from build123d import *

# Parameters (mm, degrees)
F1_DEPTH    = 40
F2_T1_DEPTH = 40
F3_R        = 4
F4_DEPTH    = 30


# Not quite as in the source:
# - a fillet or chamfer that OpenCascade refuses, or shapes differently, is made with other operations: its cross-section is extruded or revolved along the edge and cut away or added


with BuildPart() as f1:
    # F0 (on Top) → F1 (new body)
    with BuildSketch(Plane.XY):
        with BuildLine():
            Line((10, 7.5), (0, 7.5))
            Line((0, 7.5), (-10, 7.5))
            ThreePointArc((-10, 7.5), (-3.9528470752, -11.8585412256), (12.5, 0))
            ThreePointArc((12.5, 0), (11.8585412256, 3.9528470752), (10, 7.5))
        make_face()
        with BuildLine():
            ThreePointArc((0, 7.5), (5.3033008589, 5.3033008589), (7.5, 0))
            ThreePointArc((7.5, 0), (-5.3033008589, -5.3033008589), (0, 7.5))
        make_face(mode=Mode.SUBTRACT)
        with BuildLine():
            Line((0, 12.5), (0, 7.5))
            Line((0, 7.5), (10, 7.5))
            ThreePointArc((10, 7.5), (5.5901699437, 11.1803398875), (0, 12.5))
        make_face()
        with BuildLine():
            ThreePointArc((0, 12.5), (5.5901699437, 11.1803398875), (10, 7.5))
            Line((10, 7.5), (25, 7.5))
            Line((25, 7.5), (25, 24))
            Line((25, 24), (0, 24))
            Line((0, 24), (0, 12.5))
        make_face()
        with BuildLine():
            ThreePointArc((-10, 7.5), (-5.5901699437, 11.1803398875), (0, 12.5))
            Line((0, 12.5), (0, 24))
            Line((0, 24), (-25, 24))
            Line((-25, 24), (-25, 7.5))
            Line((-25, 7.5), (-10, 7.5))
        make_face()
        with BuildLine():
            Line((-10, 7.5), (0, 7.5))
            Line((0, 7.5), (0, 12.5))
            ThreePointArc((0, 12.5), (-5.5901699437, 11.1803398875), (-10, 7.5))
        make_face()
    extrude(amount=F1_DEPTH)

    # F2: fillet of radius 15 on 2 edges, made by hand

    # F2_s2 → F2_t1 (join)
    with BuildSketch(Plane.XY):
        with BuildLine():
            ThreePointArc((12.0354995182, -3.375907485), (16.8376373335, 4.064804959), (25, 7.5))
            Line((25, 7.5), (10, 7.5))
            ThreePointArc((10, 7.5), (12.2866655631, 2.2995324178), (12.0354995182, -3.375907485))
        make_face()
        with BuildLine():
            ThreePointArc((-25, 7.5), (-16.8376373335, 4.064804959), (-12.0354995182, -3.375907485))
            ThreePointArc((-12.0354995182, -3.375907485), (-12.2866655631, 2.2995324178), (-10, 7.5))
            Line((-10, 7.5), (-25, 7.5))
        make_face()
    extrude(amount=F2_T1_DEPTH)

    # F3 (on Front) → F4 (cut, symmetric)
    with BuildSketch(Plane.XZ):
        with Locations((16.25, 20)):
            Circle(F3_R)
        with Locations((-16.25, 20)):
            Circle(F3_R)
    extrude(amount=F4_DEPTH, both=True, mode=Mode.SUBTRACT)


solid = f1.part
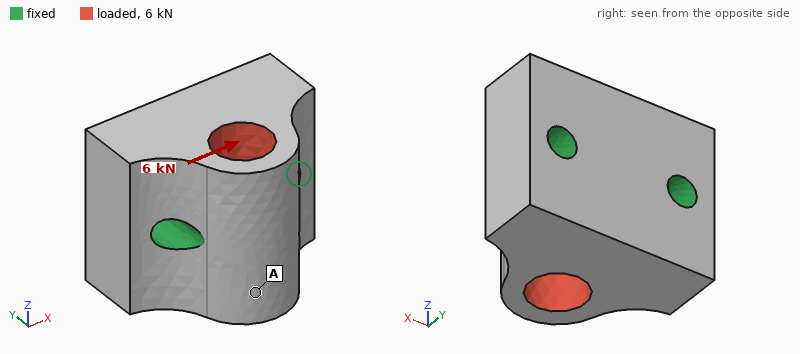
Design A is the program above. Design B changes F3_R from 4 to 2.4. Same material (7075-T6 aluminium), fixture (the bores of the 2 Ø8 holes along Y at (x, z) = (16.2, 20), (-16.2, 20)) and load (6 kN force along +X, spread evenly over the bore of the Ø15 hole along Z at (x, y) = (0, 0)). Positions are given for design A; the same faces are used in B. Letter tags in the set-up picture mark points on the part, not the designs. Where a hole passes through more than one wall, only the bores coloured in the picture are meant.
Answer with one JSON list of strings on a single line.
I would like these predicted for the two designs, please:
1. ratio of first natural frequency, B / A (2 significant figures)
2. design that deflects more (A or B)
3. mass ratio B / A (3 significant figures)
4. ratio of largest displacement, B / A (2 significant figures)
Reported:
["0.75", "B", "1.03", "1.3"]
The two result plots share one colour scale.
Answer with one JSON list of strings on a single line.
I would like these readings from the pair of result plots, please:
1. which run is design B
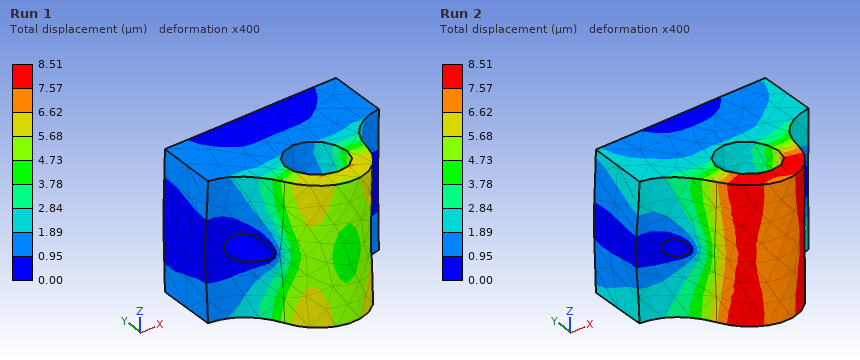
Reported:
["Run 2"]
